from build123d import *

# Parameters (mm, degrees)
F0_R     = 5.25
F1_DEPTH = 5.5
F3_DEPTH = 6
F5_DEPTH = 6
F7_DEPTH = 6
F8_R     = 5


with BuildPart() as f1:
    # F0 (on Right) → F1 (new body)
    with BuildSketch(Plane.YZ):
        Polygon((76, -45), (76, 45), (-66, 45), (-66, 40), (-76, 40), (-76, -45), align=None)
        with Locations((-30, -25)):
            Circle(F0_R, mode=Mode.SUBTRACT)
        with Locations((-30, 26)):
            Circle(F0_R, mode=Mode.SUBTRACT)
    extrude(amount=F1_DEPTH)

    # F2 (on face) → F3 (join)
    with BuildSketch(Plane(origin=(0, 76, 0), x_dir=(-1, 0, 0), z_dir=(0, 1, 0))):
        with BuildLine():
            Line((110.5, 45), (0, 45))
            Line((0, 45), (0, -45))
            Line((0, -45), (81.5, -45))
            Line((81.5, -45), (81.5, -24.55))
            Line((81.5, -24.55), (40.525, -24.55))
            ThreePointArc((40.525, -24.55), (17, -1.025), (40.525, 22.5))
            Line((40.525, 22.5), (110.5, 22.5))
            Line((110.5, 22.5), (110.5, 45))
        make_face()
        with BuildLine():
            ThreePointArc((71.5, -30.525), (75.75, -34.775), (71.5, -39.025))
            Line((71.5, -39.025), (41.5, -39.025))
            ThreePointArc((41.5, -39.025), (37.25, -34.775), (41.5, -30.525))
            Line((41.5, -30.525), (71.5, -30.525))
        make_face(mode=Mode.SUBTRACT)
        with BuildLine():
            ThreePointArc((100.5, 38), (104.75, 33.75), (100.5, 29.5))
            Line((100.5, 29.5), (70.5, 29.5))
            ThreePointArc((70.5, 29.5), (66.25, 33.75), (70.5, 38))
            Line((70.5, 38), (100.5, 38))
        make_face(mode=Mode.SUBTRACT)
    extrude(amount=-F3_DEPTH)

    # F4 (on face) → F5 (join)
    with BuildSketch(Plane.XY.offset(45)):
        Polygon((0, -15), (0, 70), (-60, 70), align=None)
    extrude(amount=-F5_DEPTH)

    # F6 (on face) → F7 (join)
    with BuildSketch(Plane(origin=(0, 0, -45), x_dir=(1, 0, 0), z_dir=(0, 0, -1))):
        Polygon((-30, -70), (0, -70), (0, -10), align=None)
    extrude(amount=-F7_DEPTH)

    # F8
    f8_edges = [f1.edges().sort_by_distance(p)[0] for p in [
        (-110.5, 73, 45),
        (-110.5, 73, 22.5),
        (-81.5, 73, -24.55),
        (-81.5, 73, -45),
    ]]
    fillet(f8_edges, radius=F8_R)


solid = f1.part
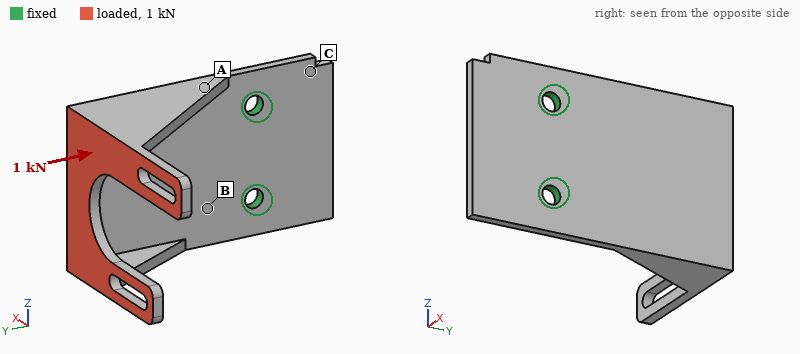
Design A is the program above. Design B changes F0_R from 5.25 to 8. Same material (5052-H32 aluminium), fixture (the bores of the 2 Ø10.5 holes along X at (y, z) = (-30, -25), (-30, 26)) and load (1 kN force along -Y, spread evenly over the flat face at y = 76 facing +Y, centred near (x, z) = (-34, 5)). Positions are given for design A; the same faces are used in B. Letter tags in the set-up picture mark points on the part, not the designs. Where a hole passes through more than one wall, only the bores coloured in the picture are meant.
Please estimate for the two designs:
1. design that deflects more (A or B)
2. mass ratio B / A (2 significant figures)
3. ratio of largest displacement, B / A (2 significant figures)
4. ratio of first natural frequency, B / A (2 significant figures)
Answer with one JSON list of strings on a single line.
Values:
["A", "0.99", "0.89", "1.1"]
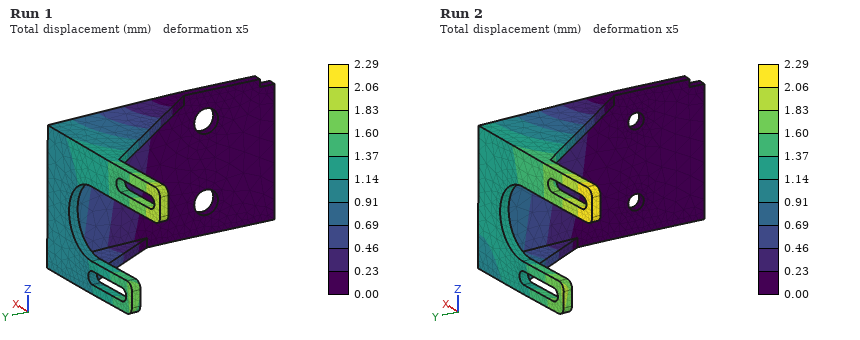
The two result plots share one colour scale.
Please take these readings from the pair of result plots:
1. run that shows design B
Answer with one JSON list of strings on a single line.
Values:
["Run 1"]
